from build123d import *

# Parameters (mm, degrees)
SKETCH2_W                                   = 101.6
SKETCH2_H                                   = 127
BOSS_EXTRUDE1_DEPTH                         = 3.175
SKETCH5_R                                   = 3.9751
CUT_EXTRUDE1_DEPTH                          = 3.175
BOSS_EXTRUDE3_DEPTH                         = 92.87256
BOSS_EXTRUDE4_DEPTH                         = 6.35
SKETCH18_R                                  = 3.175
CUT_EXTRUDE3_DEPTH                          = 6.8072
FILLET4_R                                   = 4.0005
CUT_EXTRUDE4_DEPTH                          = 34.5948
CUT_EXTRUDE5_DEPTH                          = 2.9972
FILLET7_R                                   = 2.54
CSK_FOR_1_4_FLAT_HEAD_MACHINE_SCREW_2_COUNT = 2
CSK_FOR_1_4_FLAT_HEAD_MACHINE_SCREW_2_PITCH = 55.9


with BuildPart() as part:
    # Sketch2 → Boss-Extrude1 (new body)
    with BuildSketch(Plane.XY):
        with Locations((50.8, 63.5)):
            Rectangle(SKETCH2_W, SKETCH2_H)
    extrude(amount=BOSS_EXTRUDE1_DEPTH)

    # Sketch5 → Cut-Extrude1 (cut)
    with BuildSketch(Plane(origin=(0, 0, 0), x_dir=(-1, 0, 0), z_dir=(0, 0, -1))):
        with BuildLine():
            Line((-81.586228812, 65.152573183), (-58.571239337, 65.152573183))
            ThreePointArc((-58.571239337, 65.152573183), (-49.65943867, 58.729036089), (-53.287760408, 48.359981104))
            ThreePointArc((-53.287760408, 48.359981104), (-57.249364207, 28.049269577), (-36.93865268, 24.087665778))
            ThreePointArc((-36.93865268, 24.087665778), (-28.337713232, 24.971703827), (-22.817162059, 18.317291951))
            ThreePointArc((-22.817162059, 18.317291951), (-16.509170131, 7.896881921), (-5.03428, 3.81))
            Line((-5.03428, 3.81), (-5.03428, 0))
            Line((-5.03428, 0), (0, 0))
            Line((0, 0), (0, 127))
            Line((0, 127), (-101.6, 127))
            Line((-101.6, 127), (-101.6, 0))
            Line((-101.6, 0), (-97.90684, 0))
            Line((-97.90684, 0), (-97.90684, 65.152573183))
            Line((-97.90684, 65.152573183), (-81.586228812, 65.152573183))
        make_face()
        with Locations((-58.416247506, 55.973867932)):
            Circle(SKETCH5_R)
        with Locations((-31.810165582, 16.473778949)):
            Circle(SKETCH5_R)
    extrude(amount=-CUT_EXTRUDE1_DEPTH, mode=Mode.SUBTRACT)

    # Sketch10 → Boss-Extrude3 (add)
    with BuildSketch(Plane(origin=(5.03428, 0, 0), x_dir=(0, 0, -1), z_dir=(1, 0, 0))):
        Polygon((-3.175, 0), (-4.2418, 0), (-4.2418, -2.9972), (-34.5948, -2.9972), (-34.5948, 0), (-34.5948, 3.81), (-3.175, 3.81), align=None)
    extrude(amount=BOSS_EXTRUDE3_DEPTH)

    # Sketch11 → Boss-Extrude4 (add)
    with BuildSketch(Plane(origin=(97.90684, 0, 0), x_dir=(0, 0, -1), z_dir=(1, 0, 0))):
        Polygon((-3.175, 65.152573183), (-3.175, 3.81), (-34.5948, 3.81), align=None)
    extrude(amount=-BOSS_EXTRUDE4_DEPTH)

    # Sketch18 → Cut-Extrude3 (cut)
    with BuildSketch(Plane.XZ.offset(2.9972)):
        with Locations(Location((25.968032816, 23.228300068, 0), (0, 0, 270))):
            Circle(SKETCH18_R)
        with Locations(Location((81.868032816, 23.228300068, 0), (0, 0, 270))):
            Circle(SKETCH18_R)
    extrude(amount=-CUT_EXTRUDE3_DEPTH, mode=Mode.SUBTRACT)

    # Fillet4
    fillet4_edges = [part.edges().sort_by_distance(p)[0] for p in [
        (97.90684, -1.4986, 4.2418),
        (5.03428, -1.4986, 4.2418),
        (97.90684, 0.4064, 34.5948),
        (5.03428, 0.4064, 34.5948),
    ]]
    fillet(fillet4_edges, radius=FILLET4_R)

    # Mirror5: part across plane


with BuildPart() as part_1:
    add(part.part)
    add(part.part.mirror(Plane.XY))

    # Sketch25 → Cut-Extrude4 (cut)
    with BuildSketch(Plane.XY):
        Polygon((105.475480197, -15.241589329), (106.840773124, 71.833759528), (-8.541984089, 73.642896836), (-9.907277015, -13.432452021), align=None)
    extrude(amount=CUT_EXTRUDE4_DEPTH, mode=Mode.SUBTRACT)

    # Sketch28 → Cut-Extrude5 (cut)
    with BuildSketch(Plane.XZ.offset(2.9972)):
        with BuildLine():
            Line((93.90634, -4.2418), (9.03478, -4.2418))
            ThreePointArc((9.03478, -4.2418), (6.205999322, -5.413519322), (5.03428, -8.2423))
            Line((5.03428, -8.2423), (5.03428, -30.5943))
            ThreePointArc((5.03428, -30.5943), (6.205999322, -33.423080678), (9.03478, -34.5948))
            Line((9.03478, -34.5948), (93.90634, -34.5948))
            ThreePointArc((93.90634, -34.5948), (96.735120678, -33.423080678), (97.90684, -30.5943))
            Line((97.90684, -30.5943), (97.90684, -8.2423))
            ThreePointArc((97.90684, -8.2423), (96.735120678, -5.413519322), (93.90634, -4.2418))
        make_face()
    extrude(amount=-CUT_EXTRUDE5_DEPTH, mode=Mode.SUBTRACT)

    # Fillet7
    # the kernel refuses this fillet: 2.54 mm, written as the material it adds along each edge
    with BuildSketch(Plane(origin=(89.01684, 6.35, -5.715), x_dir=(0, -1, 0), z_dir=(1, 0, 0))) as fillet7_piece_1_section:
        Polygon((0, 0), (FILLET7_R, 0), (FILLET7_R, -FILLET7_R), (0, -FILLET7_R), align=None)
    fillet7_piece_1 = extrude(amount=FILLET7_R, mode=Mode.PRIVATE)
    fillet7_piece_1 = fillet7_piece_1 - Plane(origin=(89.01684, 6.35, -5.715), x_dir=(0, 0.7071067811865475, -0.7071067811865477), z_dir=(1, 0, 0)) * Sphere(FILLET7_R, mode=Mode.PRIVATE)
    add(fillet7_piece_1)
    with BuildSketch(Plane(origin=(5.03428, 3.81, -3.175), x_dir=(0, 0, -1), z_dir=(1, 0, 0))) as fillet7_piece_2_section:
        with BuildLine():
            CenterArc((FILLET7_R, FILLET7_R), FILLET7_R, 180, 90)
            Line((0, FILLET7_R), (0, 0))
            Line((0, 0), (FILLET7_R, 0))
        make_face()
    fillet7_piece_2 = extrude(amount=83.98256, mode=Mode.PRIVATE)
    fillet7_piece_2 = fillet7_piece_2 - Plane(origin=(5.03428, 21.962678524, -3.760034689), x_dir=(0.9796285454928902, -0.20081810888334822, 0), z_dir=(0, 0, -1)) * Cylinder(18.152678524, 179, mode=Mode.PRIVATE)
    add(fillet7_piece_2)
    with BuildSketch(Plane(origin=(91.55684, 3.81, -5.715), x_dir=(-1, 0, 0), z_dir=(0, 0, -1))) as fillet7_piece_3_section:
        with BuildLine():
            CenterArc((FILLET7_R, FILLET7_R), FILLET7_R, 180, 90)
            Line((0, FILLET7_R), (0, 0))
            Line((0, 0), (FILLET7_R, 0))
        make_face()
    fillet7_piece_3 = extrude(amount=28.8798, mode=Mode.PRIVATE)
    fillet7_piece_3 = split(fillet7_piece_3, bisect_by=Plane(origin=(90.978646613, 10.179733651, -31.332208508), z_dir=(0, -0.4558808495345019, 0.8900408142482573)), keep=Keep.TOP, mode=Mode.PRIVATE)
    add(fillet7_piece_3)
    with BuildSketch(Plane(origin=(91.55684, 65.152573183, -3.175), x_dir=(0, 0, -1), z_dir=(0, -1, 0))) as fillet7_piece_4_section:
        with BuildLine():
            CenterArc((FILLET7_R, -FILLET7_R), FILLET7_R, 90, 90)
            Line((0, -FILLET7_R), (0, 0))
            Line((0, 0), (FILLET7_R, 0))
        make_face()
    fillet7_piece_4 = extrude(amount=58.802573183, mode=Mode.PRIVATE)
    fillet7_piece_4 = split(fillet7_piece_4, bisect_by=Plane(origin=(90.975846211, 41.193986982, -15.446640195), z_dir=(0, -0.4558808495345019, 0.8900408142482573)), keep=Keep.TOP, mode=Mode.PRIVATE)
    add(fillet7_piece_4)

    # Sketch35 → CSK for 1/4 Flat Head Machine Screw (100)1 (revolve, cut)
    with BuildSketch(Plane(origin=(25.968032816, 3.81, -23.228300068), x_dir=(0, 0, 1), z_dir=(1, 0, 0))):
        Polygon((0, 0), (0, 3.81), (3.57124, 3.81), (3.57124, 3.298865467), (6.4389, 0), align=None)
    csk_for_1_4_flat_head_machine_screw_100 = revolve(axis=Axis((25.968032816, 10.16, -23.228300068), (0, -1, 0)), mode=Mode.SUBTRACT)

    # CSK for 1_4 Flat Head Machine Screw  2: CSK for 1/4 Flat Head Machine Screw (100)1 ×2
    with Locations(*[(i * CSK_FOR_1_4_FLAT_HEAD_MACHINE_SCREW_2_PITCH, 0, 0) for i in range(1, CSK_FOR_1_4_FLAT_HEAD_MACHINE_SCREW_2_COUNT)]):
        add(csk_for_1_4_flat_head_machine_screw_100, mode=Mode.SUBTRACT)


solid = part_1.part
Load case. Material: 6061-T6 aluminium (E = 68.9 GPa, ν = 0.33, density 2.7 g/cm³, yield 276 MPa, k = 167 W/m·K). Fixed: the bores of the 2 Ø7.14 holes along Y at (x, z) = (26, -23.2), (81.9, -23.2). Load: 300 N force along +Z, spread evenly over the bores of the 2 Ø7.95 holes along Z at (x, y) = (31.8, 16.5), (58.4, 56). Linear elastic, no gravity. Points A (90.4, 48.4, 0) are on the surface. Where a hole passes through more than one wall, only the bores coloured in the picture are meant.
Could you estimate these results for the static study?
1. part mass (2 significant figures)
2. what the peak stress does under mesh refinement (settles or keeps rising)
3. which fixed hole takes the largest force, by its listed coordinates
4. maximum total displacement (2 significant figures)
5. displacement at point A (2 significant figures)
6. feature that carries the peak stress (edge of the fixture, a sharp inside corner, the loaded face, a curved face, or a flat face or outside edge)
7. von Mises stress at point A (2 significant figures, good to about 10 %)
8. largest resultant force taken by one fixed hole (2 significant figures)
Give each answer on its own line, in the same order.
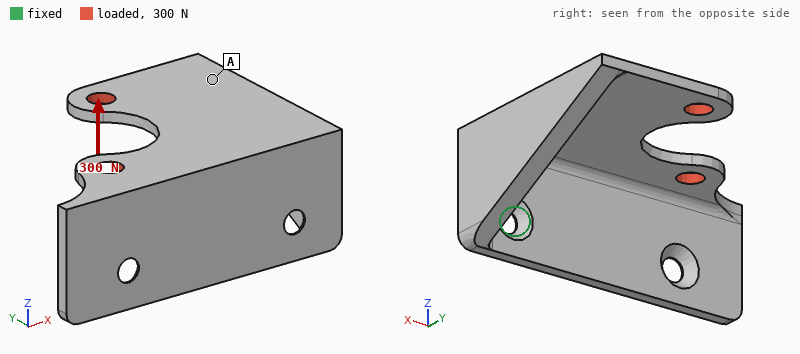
76 g
keeps rising
(26, -23.2)
1.1 mm
0.55 mm
edge of the fixture
32 MPa
220 N
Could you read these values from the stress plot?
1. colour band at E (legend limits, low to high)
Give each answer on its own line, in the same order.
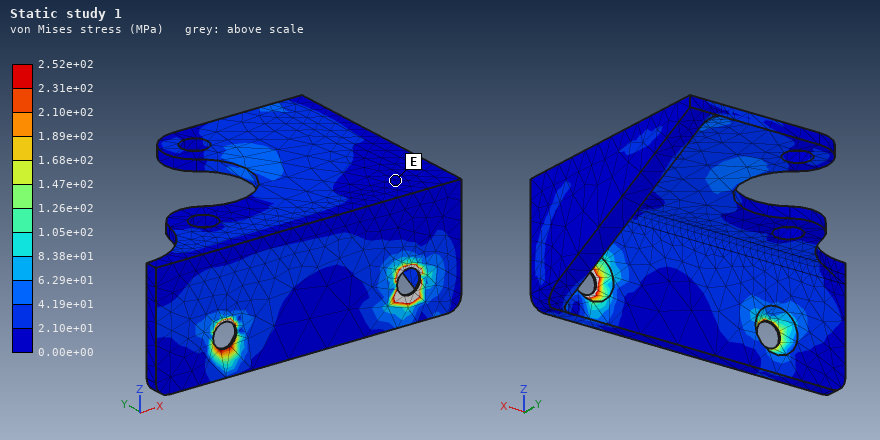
0.00e+00 to 2.10e+01 MPa
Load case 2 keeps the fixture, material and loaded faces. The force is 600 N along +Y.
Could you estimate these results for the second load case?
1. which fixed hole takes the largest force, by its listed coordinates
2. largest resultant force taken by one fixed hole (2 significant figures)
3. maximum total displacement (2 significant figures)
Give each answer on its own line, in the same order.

(26, -23.2)
400 N
0.60 mm
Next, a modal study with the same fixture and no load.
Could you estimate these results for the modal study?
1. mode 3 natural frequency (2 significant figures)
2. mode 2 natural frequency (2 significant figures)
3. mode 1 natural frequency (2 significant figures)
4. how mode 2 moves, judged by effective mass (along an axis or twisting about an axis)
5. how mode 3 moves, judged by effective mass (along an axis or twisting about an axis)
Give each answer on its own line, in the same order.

2300 Hz
1500 Hz
610 Hz
along X
along Y
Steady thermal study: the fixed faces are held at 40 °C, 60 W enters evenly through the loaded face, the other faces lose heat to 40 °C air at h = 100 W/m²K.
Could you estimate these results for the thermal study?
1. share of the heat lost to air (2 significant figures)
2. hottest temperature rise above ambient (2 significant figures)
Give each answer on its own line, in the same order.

53 %
81 K
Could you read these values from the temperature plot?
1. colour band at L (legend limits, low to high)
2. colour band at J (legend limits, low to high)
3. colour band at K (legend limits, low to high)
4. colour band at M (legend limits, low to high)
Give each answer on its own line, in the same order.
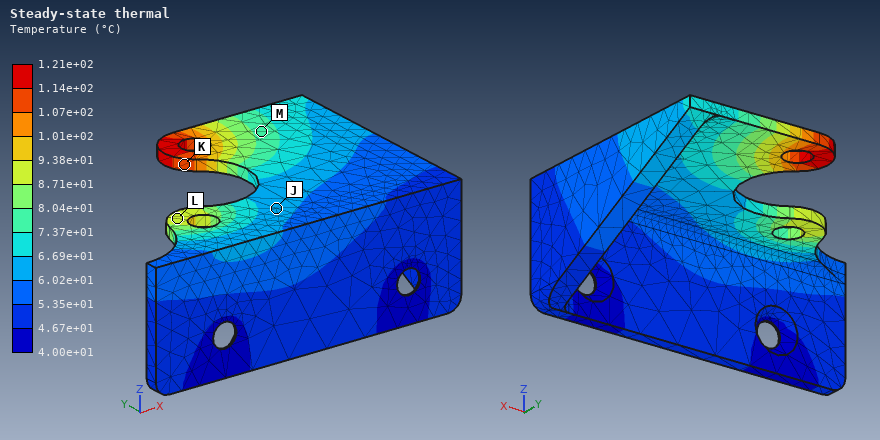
8.71e+01 to 9.38e+01 °C
6.02e+01 to 6.69e+01 °C
1.07e+02 to 1.14e+02 °C
7.37e+01 to 8.04e+01 °C
